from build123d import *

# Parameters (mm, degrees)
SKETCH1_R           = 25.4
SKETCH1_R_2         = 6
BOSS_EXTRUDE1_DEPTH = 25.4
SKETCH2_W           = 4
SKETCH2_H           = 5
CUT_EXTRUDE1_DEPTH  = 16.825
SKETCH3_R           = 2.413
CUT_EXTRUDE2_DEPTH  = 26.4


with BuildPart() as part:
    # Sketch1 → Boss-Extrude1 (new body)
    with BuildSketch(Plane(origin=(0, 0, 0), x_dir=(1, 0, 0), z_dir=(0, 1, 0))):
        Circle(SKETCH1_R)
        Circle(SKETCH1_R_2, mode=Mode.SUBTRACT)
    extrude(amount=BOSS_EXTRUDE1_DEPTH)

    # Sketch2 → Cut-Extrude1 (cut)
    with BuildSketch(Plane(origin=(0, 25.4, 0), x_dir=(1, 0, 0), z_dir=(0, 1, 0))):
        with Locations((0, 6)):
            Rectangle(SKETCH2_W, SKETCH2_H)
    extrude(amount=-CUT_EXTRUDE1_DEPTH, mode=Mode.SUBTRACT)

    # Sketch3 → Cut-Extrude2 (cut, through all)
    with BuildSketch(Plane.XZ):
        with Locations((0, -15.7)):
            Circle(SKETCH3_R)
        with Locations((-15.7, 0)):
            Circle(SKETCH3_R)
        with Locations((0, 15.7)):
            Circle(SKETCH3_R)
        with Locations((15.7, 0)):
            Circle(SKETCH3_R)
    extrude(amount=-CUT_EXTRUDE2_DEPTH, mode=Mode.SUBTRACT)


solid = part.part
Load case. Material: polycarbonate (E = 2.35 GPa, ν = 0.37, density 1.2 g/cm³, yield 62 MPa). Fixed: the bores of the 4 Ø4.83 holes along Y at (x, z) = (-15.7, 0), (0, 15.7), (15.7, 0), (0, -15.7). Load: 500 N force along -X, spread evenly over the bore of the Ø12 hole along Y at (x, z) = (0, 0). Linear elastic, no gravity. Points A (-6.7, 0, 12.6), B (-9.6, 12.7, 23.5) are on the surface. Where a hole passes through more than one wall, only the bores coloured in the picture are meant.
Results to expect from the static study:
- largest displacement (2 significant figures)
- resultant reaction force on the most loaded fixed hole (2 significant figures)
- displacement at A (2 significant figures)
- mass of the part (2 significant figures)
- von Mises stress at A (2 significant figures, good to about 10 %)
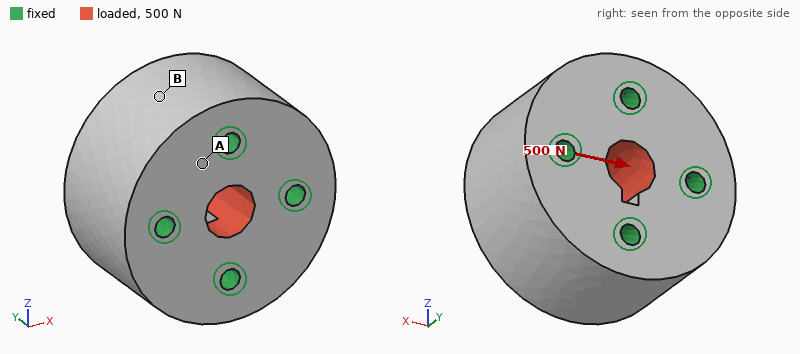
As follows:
3.0 µm
170 N
1.1 µm
56 g
0.24 MPa
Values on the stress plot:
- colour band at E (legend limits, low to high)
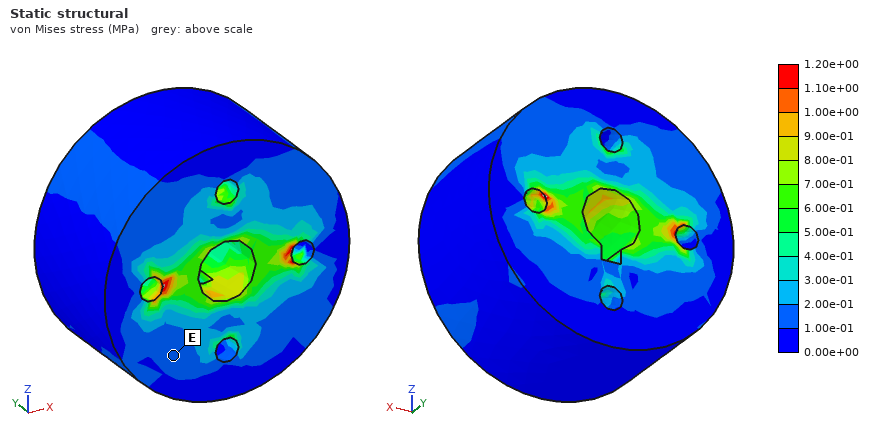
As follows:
1.00e-01 to 2.00e-01 MPa
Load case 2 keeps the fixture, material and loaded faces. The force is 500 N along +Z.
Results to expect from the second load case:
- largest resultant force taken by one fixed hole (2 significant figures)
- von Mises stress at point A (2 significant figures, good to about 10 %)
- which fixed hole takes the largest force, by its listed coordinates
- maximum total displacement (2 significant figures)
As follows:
170 N
0.25 MPa
(0, 15.7)
3.0 µm
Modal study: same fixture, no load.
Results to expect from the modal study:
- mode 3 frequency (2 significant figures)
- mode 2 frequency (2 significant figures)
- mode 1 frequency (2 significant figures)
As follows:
13 kHz
13 kHz
12 kHz
